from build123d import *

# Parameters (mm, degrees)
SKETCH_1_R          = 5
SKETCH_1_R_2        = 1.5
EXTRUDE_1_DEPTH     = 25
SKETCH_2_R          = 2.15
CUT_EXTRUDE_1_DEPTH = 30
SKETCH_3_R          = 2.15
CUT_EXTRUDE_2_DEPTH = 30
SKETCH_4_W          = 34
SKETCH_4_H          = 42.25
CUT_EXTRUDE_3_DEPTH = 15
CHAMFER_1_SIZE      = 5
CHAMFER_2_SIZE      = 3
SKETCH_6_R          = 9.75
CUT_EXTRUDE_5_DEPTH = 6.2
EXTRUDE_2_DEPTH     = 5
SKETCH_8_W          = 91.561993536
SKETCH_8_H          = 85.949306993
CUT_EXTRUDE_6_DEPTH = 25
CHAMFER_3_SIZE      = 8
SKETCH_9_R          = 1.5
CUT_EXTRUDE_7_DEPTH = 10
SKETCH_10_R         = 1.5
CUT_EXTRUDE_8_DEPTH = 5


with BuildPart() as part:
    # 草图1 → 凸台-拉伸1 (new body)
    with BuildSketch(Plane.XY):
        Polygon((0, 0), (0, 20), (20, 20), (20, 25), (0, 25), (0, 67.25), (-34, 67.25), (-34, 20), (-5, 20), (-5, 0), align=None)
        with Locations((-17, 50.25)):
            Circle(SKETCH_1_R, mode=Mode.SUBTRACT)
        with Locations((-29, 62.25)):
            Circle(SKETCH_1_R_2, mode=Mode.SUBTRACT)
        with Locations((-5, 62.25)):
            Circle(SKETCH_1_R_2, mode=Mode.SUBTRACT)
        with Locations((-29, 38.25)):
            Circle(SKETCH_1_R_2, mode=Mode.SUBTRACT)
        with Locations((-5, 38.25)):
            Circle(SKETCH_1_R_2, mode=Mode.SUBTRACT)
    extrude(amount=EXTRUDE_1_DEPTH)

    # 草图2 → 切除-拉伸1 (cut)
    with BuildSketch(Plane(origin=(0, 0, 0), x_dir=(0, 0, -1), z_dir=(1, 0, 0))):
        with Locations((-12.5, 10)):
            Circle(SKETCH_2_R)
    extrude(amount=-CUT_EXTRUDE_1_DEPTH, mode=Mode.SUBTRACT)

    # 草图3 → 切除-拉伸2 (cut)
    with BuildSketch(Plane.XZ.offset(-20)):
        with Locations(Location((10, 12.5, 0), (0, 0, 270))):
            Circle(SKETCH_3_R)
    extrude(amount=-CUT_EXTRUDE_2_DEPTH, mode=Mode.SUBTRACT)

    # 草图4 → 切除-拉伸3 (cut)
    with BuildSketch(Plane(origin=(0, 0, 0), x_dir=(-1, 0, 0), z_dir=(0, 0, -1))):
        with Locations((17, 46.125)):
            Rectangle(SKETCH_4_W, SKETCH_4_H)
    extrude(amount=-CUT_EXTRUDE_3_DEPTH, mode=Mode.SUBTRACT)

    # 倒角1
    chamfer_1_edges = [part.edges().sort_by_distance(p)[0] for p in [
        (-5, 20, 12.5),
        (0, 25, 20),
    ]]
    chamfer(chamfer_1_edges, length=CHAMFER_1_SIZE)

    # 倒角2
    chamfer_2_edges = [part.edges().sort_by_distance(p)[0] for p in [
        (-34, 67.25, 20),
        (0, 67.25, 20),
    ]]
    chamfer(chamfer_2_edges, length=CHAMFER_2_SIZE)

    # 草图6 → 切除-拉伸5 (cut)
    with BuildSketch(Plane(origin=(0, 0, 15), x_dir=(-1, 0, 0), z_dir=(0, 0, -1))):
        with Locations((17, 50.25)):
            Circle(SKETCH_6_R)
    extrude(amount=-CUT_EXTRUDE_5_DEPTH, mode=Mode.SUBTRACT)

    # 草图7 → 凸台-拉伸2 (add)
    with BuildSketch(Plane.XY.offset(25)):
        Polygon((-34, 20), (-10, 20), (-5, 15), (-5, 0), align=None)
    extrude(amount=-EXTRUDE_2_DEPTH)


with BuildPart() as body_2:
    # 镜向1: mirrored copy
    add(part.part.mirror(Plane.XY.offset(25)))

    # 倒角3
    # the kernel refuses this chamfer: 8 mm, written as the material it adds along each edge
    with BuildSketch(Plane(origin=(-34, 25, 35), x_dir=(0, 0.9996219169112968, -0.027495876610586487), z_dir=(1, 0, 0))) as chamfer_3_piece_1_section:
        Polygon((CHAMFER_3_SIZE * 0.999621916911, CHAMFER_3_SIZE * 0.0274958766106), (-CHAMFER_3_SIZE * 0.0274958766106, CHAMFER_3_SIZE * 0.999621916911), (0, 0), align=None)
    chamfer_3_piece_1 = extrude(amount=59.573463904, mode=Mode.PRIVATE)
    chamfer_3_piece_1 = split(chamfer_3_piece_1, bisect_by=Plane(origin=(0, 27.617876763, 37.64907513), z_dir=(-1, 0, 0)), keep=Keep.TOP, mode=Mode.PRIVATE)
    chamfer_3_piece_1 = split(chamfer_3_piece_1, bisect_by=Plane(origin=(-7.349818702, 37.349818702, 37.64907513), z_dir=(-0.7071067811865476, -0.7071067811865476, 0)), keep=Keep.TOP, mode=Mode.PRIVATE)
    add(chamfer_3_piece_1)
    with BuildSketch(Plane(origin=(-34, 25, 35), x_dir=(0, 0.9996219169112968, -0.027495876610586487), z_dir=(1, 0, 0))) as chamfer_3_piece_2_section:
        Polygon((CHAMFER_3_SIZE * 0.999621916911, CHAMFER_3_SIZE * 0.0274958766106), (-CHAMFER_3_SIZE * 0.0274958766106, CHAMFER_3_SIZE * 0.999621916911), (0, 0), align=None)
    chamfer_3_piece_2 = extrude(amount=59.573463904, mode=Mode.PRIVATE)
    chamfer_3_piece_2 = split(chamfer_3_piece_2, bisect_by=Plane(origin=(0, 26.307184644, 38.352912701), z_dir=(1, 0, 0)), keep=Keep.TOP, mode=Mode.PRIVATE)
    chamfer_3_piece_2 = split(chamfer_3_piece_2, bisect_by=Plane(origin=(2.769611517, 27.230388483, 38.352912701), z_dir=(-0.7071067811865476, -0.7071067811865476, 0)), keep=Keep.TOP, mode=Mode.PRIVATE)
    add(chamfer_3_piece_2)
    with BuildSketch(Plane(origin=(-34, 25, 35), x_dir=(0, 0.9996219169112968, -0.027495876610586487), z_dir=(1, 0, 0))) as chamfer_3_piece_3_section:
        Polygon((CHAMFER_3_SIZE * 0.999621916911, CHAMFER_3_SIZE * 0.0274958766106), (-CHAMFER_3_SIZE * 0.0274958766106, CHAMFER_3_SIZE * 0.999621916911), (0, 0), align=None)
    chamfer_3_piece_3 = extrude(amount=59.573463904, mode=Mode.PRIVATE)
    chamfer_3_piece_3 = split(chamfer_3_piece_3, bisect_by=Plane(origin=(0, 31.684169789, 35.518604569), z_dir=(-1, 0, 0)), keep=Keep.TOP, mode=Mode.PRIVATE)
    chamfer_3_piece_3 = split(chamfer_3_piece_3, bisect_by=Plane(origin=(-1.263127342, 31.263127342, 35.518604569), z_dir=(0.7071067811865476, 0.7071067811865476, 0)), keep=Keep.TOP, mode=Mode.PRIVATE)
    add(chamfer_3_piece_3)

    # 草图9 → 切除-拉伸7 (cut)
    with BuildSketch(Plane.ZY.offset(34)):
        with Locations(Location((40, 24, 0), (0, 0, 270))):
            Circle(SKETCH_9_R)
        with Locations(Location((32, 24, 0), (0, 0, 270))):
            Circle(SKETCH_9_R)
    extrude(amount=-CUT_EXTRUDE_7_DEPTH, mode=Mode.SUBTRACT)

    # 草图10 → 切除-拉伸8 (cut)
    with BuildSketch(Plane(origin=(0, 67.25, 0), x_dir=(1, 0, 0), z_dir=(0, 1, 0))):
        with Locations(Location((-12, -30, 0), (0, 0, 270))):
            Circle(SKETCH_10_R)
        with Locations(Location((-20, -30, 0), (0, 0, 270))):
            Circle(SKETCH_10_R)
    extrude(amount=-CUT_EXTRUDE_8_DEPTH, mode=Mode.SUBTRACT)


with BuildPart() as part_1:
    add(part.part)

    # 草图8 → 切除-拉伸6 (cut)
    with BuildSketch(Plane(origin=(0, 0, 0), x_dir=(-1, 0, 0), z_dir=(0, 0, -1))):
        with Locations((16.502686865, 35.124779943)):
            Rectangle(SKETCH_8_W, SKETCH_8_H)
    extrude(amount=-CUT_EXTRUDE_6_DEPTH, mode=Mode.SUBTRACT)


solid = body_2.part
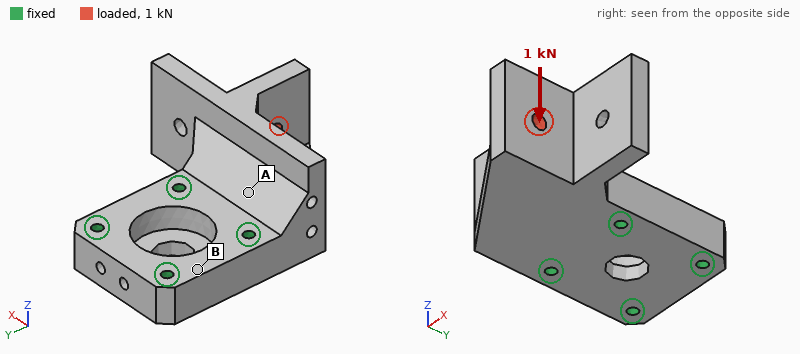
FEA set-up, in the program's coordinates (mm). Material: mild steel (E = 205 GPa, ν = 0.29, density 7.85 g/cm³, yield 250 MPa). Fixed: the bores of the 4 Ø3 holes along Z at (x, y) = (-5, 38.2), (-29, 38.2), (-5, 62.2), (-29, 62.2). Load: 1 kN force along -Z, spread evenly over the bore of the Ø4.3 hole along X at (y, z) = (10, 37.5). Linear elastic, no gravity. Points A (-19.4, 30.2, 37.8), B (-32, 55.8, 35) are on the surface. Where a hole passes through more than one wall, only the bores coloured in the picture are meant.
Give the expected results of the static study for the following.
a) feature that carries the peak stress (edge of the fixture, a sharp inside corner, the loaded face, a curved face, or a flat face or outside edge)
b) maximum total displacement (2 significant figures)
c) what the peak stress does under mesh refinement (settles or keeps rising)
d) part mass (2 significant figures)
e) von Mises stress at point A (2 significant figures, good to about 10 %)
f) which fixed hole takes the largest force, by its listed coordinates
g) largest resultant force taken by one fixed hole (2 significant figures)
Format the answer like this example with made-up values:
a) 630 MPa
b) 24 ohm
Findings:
a) edge of the fixture
b) 31 µm
c) keeps rising
d) 190 g
e) 22 MPa
f) (-5, 38.2)
g) 1.1 kN
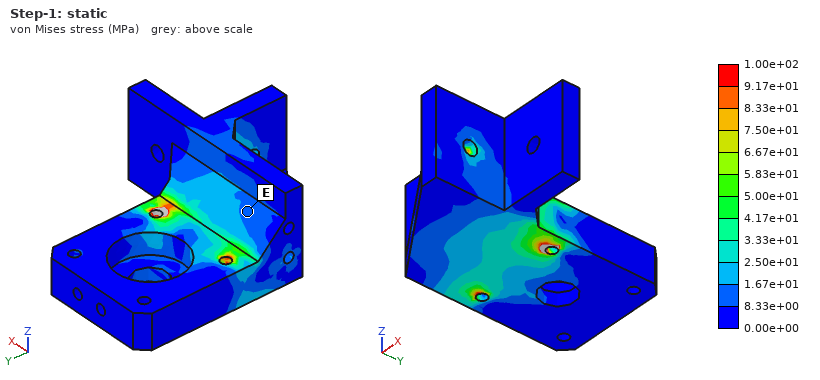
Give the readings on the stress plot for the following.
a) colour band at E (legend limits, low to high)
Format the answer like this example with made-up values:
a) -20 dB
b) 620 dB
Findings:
a) 8.33e+00 to 1.67e+01 MPa
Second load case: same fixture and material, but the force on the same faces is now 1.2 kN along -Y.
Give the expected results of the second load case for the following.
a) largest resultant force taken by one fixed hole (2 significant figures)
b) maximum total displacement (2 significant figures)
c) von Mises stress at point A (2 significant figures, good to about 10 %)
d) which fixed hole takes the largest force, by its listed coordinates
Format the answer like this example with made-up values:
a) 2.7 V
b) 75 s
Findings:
a) 1.2 kN
b) 11 µm
c) 7.3 MPa
d) (-5, 38.2)
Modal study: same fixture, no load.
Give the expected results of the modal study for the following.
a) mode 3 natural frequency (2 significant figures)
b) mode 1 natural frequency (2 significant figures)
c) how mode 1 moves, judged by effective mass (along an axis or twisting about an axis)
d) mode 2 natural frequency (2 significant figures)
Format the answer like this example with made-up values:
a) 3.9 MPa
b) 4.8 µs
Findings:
a) 10 kHz
b) 5000 Hz
c) along Z
d) 9000 Hz
